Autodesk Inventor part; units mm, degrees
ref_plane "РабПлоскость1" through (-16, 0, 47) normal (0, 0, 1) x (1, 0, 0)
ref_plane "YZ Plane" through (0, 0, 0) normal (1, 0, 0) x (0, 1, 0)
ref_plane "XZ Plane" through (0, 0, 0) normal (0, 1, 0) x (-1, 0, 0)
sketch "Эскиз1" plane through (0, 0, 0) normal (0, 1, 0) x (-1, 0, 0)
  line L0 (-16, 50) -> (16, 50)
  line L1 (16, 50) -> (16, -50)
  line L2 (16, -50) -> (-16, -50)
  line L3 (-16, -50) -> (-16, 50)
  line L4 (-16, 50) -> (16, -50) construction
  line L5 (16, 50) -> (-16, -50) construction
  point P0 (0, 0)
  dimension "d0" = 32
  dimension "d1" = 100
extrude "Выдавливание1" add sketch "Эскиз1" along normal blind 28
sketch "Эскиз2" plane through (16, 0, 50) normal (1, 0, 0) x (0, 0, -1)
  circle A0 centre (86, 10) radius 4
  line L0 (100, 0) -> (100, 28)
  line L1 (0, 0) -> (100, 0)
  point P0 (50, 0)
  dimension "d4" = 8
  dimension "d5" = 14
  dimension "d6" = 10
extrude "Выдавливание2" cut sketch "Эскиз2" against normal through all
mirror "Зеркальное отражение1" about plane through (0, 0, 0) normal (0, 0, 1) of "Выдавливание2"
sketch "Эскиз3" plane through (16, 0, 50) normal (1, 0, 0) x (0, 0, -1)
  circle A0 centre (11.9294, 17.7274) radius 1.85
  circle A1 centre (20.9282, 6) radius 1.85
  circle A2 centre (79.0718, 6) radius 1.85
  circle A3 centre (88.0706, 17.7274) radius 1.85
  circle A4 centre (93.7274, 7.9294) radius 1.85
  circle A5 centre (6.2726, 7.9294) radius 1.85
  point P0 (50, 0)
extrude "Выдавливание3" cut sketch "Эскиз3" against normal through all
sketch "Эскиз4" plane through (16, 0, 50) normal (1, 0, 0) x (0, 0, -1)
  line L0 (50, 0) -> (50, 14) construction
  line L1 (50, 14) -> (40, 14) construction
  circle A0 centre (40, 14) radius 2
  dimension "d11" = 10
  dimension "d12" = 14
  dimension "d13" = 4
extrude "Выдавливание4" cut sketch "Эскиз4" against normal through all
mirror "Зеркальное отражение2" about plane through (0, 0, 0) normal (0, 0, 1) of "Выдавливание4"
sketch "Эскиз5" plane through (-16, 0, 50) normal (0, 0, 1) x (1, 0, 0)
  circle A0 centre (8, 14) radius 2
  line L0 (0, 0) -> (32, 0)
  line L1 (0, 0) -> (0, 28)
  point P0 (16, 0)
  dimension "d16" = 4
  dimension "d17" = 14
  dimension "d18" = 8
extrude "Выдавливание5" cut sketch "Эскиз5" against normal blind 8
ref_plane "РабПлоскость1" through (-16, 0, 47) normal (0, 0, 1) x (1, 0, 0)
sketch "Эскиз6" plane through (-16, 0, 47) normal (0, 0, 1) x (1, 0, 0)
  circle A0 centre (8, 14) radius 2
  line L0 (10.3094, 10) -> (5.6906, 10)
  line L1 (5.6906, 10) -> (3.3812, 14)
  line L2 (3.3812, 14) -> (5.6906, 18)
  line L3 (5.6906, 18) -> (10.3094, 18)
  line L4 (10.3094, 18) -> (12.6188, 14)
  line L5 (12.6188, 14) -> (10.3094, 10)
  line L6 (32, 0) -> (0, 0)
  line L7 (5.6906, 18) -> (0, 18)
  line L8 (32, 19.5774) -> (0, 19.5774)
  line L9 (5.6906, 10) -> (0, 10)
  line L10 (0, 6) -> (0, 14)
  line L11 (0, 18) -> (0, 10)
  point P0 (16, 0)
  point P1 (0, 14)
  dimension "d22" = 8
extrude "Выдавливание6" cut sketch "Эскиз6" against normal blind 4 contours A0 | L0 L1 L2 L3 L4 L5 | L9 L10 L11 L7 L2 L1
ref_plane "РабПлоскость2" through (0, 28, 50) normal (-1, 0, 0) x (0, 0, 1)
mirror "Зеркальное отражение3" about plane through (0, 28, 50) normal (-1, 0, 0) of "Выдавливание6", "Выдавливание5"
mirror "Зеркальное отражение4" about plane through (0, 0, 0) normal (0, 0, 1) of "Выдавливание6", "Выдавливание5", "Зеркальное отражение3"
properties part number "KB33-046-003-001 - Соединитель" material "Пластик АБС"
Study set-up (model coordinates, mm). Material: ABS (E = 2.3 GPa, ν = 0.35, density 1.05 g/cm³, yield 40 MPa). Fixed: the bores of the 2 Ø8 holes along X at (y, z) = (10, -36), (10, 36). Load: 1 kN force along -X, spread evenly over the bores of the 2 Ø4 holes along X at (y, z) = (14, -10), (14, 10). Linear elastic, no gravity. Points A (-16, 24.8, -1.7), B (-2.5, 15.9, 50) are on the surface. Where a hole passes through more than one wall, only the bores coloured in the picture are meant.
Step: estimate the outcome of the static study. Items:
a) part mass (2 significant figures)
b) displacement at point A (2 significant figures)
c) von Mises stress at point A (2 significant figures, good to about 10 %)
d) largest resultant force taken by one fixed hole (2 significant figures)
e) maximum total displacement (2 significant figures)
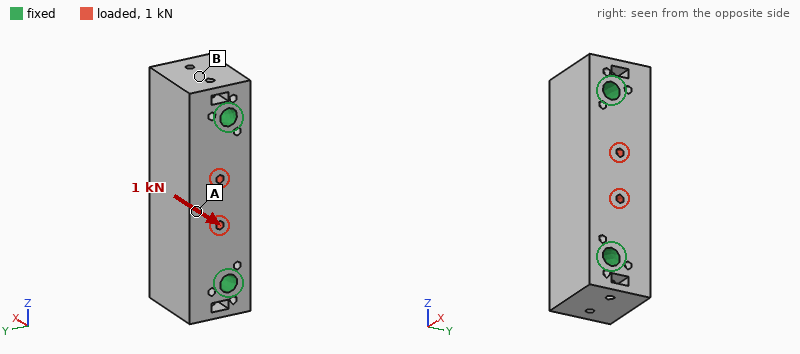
86 g
31 µm
1.3 MPa
500 N
36 µm
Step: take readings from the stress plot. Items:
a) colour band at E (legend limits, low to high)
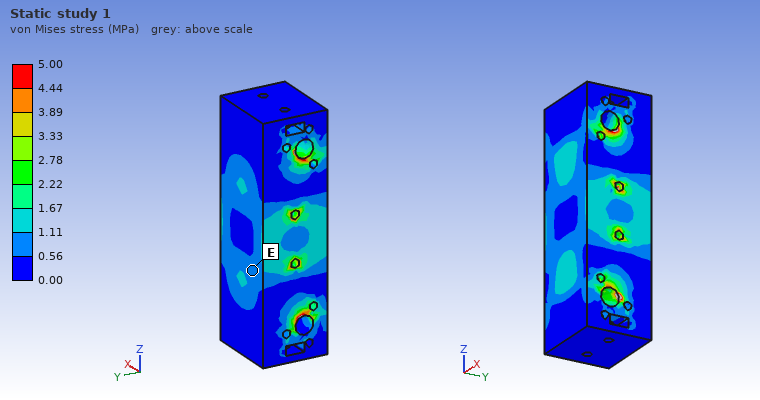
0.56 to 1.11 MPa
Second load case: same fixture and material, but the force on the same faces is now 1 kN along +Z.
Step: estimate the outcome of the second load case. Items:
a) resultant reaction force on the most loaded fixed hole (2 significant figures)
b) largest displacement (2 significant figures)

500 N
11 µm
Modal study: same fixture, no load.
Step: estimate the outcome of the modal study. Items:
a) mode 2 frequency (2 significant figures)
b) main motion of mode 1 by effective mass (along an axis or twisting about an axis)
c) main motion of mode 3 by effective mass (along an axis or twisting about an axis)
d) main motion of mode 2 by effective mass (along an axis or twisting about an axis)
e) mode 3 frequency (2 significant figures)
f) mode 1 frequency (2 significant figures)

4600 Hz
along Y
twisting about Z
along X
5400 Hz
3900 Hz
